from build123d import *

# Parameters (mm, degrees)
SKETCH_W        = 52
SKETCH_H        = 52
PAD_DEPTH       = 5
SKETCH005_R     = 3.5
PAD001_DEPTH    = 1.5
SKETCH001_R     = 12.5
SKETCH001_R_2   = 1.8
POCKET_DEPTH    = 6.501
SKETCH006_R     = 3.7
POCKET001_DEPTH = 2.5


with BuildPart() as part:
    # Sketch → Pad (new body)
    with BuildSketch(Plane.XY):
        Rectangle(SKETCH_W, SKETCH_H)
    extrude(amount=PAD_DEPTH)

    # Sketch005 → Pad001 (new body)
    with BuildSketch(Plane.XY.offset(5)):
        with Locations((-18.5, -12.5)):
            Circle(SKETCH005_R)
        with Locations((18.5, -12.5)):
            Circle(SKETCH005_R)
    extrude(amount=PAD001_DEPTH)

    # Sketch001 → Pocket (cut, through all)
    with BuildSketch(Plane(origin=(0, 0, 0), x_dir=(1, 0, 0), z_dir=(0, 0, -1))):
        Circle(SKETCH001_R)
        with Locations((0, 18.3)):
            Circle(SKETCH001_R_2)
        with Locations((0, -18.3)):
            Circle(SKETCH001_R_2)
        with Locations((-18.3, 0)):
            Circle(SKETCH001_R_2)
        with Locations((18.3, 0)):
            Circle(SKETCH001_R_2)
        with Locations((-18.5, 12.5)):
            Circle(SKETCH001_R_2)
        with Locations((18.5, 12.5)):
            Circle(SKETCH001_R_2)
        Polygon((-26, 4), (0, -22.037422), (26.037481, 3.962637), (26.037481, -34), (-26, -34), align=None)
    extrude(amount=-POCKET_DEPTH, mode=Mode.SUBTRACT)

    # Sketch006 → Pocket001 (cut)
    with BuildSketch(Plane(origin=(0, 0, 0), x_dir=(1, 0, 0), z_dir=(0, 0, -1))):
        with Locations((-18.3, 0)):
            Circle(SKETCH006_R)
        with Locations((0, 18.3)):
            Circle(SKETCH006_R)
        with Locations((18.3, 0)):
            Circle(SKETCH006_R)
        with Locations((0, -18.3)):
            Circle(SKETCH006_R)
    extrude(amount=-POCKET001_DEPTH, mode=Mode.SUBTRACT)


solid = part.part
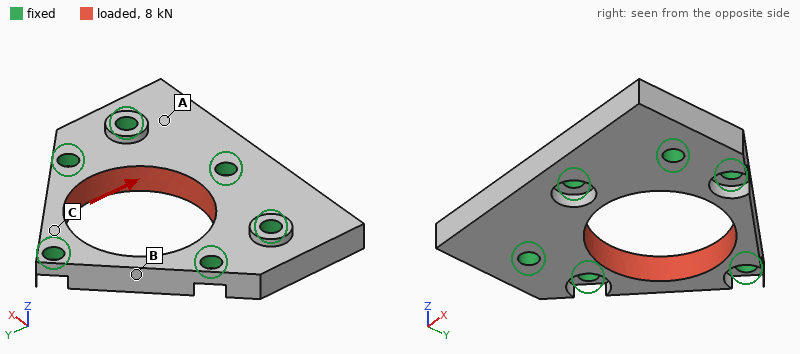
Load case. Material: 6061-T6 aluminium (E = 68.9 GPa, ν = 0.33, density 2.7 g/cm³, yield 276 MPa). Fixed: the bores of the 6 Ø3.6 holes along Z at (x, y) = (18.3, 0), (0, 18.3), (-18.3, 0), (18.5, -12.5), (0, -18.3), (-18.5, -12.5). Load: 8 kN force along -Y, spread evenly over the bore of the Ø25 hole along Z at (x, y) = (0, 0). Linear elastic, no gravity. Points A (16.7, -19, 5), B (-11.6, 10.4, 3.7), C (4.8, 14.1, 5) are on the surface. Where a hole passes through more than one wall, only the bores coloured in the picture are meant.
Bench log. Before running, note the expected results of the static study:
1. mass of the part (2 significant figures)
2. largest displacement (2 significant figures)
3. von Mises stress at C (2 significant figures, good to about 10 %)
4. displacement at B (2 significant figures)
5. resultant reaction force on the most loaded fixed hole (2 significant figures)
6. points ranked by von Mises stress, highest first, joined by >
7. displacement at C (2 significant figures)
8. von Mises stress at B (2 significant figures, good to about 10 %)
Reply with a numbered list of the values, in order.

1. 17 g
2. 26 µm
3. 61 MPa
4. 21 µm
5. 1.6 kN
6. B > C > A
7. 7.6 µm
8. 95 MPa
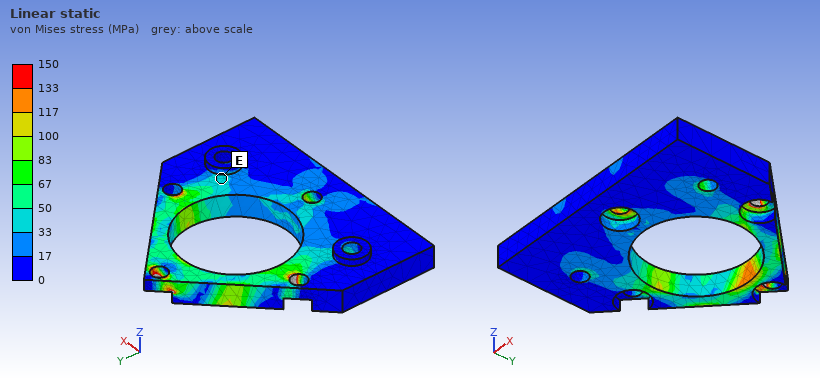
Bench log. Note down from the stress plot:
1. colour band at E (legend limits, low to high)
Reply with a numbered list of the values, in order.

1. 33 to 50 MPa
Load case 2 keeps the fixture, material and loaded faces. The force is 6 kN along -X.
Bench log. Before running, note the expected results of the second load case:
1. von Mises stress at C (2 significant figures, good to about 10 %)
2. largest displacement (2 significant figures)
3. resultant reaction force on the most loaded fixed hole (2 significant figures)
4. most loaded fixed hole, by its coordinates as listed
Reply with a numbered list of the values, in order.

1. 58 MPa
2. 33 µm
3. 1.7 kN
4. (0, 18.3)
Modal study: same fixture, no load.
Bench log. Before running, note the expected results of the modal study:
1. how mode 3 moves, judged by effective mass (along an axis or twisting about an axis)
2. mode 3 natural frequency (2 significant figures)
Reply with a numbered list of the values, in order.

1. along Z
2. 23 kHz
